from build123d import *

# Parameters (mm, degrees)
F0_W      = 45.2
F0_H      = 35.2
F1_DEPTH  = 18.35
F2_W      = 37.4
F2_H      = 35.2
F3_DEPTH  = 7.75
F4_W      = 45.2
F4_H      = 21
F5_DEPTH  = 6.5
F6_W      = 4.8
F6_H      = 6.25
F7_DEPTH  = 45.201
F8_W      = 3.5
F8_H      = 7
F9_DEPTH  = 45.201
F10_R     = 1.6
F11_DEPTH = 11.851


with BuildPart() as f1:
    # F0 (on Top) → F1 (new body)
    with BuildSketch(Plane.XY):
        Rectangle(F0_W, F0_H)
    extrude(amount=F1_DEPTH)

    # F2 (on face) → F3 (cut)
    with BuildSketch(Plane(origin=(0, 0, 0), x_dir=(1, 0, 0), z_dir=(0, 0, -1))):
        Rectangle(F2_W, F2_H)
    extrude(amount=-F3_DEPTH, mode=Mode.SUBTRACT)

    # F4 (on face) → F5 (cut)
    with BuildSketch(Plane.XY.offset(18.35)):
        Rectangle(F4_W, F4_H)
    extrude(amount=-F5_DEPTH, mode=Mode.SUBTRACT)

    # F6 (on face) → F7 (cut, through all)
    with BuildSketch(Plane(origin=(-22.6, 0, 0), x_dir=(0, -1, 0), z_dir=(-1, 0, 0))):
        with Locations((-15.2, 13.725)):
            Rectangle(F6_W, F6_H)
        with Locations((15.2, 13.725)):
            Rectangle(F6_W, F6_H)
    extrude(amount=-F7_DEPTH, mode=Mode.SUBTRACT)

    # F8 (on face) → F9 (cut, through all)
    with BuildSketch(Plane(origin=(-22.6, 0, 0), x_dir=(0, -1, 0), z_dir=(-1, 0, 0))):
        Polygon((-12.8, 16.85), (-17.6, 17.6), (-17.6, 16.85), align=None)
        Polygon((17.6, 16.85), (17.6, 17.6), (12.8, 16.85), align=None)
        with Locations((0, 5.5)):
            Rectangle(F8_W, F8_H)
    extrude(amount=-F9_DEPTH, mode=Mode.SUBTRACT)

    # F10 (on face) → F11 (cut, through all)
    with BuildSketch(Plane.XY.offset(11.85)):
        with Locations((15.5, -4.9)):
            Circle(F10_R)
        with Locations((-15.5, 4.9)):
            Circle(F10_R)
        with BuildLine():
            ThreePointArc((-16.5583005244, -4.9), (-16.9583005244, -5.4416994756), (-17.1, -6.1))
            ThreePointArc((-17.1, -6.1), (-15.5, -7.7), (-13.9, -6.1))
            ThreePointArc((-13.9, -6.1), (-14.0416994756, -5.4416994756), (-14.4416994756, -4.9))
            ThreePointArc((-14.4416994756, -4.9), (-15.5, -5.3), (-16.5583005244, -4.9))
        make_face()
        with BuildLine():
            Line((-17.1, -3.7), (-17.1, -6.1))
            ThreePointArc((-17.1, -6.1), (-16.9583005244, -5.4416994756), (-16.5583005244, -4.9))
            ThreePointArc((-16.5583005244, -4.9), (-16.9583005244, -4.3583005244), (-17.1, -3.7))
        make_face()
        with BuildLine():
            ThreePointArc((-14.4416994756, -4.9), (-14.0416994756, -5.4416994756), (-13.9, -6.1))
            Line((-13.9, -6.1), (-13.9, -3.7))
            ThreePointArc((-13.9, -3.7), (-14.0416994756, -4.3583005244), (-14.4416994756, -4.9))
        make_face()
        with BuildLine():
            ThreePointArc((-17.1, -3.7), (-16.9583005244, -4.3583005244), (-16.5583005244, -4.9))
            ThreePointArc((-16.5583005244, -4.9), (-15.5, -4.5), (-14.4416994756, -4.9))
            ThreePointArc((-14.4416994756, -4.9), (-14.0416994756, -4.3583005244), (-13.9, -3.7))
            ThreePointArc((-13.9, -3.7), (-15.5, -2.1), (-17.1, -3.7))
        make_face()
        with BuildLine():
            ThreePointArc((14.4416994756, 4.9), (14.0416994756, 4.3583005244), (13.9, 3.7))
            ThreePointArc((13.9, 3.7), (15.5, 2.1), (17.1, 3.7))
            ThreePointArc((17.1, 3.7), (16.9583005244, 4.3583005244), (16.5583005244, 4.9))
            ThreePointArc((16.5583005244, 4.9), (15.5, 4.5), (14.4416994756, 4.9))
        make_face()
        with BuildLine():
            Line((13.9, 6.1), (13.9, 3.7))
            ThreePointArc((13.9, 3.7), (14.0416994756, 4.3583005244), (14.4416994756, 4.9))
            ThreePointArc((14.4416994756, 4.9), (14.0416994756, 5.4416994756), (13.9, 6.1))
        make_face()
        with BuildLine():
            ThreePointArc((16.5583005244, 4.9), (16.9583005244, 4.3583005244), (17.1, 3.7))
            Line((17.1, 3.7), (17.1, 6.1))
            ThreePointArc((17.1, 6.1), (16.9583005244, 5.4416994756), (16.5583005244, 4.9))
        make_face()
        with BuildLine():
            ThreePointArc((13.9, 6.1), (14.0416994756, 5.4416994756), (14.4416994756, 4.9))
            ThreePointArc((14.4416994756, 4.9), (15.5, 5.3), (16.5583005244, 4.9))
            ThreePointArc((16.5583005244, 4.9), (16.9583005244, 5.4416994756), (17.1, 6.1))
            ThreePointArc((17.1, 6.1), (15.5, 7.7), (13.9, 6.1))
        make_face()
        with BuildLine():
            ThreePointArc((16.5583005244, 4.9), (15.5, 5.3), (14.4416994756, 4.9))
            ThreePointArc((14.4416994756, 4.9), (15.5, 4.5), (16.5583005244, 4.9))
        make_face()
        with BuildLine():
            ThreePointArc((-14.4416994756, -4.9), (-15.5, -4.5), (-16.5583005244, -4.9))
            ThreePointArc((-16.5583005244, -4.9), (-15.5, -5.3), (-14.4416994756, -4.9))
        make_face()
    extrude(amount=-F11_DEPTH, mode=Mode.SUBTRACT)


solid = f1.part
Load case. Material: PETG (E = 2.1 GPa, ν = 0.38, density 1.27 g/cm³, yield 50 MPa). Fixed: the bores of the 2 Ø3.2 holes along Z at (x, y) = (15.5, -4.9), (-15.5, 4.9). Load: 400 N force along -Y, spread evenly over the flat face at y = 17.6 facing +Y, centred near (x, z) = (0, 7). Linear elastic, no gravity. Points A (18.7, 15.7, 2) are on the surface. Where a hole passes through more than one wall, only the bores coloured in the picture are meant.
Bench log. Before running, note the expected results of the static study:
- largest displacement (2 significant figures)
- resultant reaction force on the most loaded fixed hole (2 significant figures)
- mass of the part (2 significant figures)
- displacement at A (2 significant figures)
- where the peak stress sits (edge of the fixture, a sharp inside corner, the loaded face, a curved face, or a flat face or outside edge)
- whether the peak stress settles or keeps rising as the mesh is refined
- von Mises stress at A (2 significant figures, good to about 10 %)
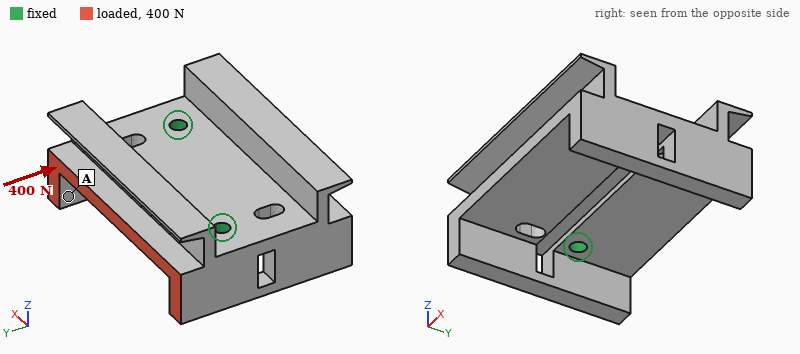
0.23 mm
200 N
12 g
0.20 mm
edge of the fixture
keeps rising
2.1 MPa
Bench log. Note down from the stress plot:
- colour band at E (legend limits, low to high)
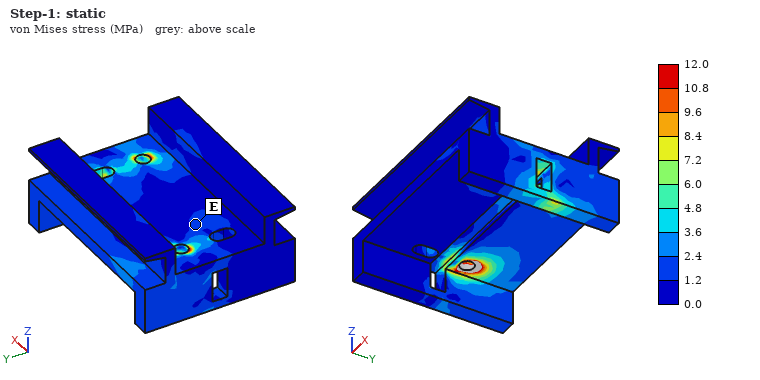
1.2 to 2.4 MPa
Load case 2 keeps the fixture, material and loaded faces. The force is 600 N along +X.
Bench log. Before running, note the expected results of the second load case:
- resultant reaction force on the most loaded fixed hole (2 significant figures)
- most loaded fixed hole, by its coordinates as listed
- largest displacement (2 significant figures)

530 N
(-15.5, 4.9)
0.64 mm
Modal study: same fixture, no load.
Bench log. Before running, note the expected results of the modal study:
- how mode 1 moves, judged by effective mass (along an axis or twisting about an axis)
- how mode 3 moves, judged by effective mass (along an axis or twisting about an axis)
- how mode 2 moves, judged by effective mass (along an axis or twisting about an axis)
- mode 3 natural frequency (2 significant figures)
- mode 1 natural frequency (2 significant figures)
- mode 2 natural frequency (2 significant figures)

twisting about X
along Z
along Z
3500 Hz
1400 Hz
1700 Hz
